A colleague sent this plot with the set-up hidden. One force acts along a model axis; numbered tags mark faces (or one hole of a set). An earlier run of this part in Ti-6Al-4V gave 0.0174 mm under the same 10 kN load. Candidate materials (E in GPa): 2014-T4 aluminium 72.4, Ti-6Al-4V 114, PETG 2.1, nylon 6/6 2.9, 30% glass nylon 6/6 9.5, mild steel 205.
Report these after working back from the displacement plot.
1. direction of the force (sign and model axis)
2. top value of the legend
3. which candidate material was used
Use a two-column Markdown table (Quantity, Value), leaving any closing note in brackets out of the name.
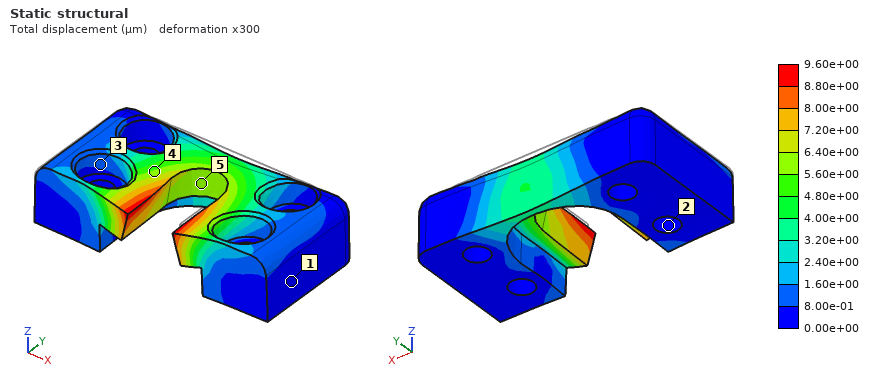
| Quantity | Value |
|---|---|
| direction of the force | -Z |
| top value of the legend | 9.60e+00 µm |
| which candidate material was used | mild steel |
